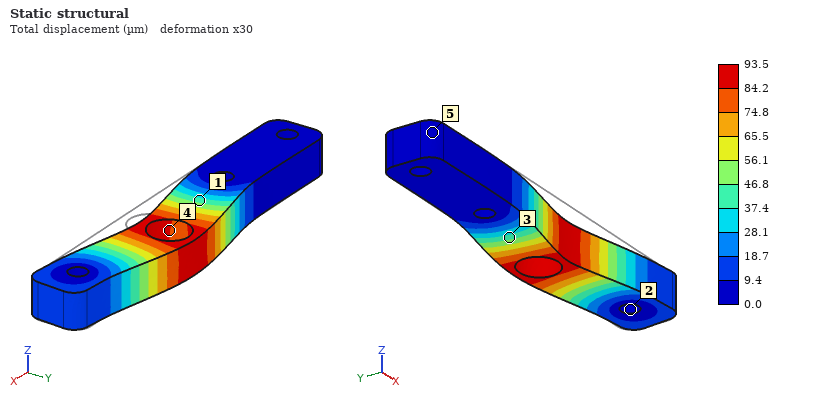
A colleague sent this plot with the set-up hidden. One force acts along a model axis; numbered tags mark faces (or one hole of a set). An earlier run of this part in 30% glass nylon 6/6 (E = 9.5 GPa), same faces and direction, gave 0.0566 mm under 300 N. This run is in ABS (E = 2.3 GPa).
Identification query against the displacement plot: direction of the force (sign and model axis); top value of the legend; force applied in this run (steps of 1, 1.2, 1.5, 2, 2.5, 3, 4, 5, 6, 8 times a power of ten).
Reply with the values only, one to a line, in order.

+Y
93.5 µm
120 N
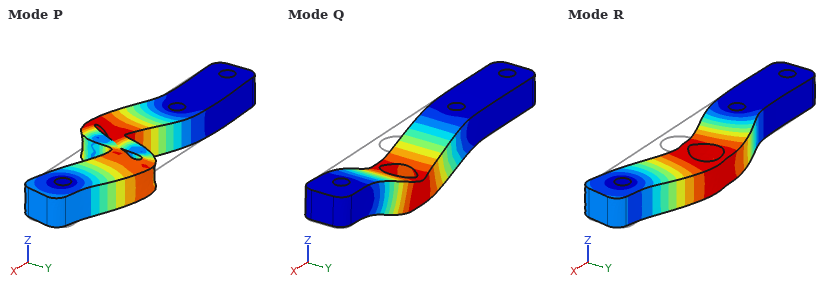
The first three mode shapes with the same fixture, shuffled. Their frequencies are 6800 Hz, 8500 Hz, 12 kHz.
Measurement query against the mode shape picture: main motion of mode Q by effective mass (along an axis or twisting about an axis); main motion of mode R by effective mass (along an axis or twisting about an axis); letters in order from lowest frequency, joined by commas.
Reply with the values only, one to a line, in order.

along Z
along Y
Q, R, P
